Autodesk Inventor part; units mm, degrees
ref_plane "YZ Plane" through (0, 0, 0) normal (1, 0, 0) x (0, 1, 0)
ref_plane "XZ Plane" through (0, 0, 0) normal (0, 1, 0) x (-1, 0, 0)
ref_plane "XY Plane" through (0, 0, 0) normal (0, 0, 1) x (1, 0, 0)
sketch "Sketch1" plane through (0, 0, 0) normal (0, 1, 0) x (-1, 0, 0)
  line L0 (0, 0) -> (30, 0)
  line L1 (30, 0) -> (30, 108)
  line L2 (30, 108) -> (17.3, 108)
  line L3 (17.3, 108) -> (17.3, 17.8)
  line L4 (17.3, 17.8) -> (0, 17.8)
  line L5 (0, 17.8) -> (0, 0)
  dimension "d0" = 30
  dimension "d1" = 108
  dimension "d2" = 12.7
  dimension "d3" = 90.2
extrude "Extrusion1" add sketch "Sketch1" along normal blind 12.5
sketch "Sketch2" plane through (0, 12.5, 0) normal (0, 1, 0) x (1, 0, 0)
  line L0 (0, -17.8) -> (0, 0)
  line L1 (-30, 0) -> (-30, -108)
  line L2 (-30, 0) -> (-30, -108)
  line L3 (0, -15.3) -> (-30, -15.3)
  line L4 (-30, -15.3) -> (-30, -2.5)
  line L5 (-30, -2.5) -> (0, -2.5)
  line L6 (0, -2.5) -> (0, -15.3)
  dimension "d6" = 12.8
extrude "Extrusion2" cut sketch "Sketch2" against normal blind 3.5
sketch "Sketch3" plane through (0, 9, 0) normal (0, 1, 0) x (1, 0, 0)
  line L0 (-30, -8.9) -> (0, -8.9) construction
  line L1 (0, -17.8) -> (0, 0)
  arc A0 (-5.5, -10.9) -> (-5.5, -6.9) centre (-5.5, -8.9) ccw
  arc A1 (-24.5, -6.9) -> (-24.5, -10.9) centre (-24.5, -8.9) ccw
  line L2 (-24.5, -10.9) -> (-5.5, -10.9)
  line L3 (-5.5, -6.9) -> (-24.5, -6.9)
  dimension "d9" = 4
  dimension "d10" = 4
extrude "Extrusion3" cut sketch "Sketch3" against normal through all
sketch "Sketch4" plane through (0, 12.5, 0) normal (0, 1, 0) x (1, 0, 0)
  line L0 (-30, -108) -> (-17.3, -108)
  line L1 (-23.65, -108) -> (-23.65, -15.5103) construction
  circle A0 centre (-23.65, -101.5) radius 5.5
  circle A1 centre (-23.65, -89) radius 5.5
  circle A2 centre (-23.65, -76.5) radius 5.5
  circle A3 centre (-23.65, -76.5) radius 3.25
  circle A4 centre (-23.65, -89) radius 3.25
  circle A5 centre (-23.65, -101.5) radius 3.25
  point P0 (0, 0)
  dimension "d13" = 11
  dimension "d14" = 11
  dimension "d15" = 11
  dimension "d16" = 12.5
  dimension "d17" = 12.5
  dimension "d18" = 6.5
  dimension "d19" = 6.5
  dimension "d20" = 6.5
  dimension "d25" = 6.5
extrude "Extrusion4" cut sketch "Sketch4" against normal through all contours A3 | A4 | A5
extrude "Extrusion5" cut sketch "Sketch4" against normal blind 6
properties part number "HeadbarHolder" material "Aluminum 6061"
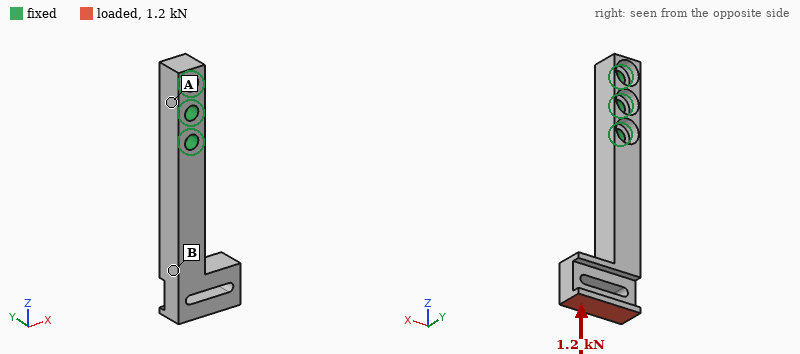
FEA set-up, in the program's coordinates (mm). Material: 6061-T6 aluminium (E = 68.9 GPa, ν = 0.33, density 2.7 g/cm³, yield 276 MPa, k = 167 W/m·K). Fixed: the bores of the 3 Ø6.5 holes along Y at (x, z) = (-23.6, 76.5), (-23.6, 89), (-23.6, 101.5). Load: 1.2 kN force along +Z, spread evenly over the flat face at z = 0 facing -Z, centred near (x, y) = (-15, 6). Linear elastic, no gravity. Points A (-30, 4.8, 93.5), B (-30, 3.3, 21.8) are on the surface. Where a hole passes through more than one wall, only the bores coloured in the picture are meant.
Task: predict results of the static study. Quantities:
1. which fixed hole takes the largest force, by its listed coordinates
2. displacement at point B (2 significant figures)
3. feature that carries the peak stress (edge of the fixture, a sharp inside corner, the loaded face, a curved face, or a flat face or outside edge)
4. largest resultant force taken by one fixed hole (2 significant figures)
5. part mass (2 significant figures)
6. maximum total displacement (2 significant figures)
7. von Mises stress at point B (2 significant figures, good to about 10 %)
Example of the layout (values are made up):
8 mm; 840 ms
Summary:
(-23.6, 76.5); 0.13 mm; a curved face; 1.0 kN; 45 g; 0.32 mm; 26 MPa
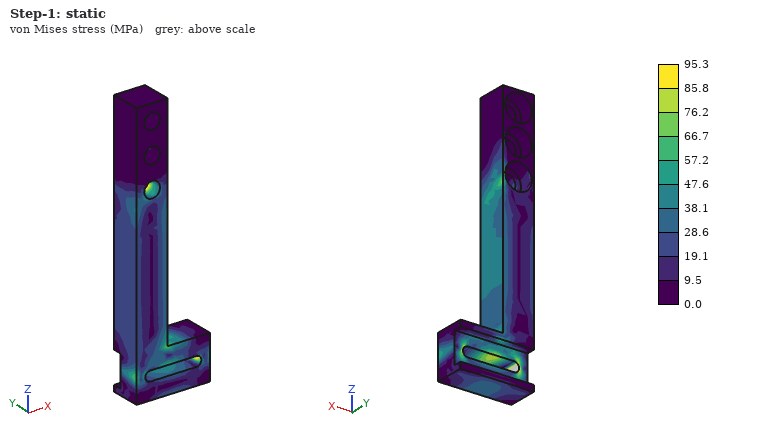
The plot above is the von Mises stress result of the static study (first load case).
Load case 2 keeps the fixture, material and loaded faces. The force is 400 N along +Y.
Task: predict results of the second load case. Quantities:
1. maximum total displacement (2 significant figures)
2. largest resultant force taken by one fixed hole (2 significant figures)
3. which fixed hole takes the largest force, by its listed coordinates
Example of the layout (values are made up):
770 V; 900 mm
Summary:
0.72 mm; 1.3 kN; (-23.6, 76.5)
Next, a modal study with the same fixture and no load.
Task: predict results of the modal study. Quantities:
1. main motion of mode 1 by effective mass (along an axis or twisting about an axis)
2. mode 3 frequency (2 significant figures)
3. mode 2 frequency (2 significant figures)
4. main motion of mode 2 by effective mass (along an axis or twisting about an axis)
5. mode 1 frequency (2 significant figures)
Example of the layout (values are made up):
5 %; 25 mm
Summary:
along Y; 4400 Hz; 1300 Hz; along X; 1100 Hz
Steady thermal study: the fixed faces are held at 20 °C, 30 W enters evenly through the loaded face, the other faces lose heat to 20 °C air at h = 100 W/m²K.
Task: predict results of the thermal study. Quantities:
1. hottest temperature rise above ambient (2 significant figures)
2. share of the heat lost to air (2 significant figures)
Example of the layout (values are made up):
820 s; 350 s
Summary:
69 K; 54 %
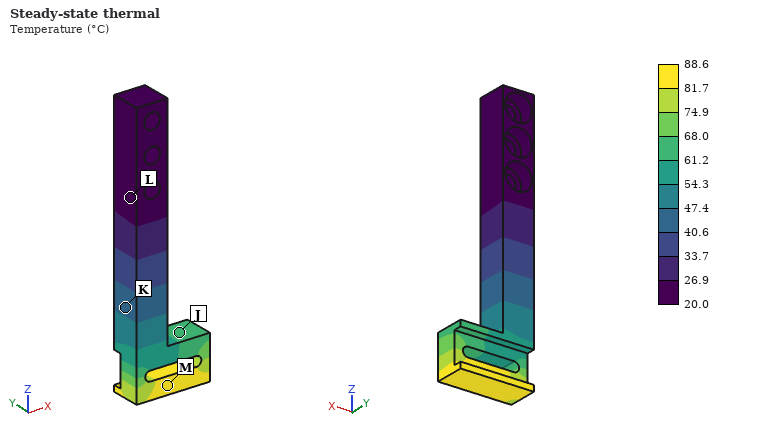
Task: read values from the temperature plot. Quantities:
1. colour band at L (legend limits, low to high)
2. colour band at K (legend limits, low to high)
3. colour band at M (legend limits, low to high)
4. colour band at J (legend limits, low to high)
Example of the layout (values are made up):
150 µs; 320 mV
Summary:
20.0 to 26.9 °C; 40.6 to 47.4 °C; 81.7 to 88.6 °C; 61.2 to 68.0 °C
